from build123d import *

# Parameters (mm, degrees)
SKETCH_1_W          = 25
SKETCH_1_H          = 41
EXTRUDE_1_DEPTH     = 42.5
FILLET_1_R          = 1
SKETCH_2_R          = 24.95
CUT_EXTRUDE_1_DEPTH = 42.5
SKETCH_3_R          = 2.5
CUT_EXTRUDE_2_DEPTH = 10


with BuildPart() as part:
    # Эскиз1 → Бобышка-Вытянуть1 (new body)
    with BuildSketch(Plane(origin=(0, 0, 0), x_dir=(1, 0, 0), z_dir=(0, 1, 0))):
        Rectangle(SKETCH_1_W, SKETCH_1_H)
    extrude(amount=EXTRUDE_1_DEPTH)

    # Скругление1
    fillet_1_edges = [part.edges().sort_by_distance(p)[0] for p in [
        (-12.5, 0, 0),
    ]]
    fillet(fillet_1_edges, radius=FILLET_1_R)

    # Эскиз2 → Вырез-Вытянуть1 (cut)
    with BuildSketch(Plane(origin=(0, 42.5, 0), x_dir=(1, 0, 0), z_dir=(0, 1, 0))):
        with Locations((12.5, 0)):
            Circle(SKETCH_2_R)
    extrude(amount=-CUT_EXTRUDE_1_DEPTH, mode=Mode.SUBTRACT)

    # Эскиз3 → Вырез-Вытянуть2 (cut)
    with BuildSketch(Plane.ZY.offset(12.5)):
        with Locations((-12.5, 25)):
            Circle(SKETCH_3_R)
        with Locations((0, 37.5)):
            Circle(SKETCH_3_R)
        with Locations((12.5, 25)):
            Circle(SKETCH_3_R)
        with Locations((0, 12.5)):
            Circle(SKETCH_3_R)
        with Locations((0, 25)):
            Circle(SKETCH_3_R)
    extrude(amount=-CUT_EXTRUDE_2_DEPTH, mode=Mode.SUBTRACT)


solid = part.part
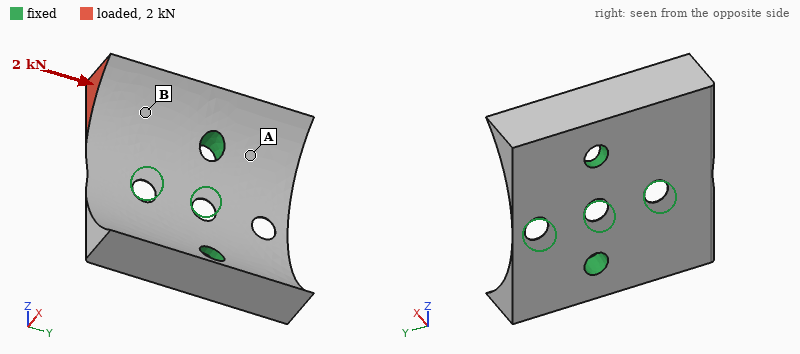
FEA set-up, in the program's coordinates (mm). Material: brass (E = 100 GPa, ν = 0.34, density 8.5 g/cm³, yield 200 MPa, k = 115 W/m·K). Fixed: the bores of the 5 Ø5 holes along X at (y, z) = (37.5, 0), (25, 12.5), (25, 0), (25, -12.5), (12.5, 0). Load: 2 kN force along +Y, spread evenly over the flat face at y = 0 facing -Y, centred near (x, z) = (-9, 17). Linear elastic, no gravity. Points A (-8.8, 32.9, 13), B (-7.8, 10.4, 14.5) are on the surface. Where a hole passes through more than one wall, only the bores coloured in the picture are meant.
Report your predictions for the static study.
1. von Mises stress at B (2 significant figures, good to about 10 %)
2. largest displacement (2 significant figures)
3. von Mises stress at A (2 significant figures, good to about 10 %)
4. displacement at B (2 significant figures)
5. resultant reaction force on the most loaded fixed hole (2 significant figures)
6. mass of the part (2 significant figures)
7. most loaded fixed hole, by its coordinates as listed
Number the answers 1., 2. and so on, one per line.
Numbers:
1. 40 MPa
2. 34 µm
3. 15 MPa
4. 14 µm
5. 2.1 kN
6. 47 g
7. (25, 12.5)
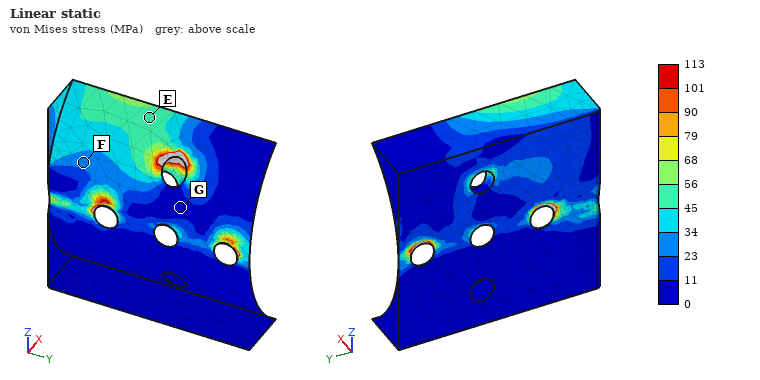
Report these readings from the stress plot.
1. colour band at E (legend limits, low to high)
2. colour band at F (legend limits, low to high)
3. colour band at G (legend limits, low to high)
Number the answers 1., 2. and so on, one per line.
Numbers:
1. 45 to 56 MPa
2. 23 to 34 MPa
3. 0 to 11 MPa
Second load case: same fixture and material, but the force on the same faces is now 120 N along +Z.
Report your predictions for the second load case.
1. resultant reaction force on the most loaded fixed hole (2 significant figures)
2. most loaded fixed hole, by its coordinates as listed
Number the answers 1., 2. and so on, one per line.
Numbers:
1. 94 N
2. (12.5, 0)
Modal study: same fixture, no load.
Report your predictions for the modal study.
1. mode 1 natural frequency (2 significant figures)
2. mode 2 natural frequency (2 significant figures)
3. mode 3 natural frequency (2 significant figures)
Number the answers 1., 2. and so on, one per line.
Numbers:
1. 4700 Hz
2. 4800 Hz
3. 9700 Hz
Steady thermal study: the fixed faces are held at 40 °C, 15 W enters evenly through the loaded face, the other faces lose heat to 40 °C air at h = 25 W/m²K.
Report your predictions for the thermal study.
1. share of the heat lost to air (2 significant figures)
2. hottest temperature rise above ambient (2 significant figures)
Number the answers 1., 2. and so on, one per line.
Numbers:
1. 5.0 %
2. 49 K
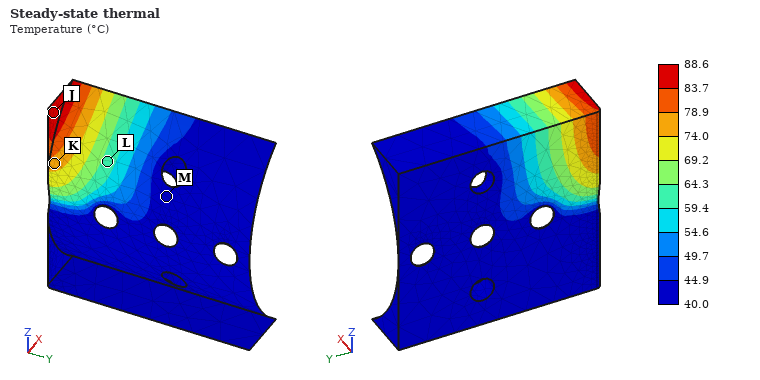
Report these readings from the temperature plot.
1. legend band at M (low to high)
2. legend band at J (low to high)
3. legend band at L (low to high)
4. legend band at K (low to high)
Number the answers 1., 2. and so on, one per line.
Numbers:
1. 40.0 to 44.9 °C
2. 83.7 to 88.6 °C
3. 59.4 to 64.3 °C
4. 74.0 to 78.9 °C
